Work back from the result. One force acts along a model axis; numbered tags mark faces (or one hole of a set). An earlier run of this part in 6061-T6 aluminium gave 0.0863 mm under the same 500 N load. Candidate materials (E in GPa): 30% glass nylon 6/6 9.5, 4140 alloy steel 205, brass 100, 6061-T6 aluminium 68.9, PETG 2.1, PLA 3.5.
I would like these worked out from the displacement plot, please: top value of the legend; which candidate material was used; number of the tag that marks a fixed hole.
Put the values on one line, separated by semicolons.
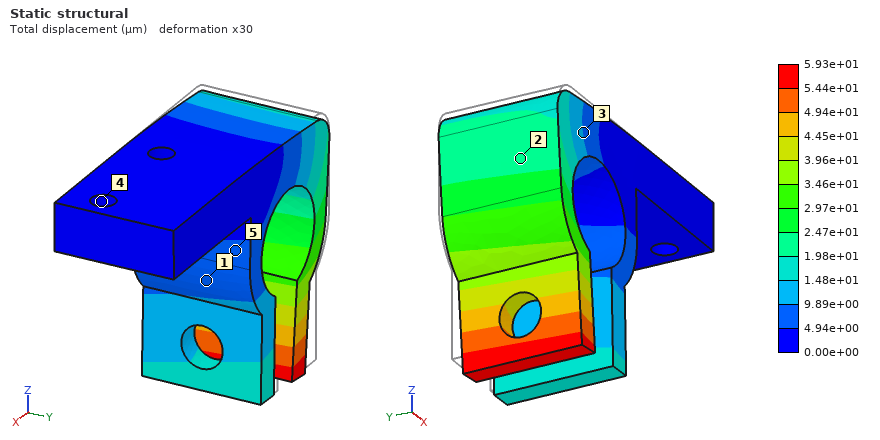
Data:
5.93e+01 µm; brass; 4
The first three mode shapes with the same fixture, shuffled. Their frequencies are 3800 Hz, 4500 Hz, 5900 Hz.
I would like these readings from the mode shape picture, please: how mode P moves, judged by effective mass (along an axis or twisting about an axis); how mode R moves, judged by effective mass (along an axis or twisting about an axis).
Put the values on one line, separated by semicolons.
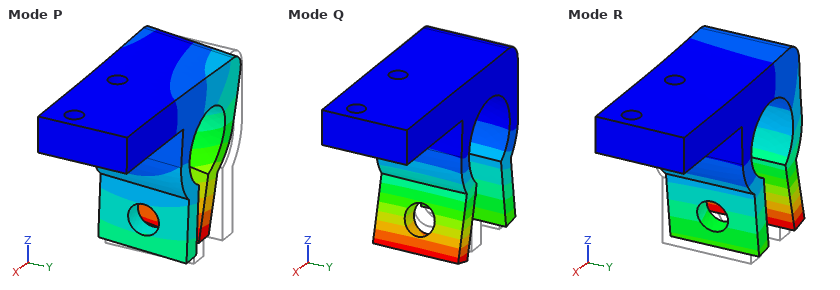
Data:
along Y; along X
